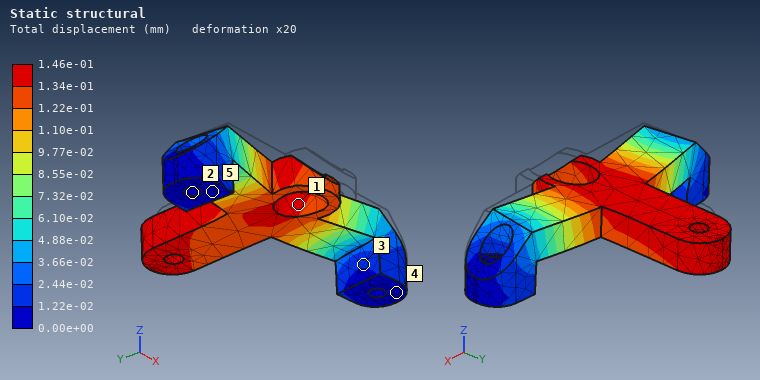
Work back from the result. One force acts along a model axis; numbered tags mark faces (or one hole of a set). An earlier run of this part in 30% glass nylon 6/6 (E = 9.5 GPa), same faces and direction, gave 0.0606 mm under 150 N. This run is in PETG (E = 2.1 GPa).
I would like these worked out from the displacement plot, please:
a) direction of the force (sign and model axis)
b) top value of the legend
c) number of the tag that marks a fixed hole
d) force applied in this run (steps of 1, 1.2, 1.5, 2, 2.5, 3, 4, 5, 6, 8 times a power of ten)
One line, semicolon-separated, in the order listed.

+Y; 1.46e-01 mm; 2; 80 N
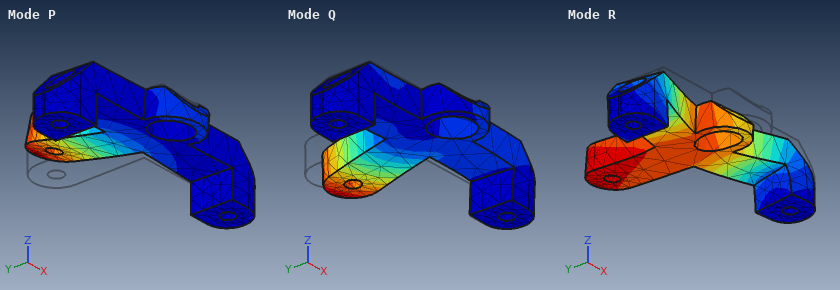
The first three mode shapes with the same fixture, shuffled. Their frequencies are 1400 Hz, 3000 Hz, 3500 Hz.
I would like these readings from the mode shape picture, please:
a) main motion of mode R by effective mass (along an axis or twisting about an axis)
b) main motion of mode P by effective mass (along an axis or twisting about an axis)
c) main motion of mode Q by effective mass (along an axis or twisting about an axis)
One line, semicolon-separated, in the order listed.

along Y; along Z; along X
